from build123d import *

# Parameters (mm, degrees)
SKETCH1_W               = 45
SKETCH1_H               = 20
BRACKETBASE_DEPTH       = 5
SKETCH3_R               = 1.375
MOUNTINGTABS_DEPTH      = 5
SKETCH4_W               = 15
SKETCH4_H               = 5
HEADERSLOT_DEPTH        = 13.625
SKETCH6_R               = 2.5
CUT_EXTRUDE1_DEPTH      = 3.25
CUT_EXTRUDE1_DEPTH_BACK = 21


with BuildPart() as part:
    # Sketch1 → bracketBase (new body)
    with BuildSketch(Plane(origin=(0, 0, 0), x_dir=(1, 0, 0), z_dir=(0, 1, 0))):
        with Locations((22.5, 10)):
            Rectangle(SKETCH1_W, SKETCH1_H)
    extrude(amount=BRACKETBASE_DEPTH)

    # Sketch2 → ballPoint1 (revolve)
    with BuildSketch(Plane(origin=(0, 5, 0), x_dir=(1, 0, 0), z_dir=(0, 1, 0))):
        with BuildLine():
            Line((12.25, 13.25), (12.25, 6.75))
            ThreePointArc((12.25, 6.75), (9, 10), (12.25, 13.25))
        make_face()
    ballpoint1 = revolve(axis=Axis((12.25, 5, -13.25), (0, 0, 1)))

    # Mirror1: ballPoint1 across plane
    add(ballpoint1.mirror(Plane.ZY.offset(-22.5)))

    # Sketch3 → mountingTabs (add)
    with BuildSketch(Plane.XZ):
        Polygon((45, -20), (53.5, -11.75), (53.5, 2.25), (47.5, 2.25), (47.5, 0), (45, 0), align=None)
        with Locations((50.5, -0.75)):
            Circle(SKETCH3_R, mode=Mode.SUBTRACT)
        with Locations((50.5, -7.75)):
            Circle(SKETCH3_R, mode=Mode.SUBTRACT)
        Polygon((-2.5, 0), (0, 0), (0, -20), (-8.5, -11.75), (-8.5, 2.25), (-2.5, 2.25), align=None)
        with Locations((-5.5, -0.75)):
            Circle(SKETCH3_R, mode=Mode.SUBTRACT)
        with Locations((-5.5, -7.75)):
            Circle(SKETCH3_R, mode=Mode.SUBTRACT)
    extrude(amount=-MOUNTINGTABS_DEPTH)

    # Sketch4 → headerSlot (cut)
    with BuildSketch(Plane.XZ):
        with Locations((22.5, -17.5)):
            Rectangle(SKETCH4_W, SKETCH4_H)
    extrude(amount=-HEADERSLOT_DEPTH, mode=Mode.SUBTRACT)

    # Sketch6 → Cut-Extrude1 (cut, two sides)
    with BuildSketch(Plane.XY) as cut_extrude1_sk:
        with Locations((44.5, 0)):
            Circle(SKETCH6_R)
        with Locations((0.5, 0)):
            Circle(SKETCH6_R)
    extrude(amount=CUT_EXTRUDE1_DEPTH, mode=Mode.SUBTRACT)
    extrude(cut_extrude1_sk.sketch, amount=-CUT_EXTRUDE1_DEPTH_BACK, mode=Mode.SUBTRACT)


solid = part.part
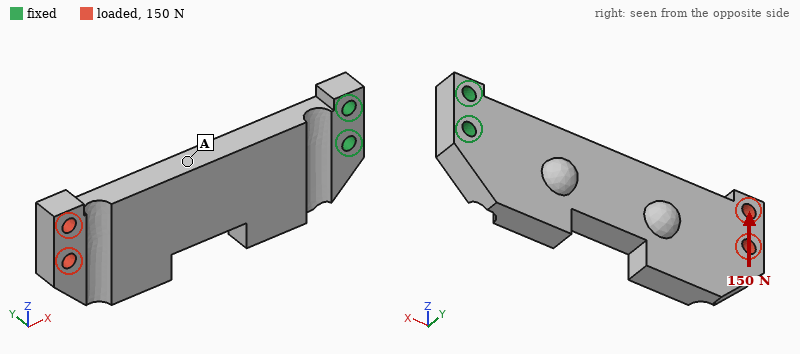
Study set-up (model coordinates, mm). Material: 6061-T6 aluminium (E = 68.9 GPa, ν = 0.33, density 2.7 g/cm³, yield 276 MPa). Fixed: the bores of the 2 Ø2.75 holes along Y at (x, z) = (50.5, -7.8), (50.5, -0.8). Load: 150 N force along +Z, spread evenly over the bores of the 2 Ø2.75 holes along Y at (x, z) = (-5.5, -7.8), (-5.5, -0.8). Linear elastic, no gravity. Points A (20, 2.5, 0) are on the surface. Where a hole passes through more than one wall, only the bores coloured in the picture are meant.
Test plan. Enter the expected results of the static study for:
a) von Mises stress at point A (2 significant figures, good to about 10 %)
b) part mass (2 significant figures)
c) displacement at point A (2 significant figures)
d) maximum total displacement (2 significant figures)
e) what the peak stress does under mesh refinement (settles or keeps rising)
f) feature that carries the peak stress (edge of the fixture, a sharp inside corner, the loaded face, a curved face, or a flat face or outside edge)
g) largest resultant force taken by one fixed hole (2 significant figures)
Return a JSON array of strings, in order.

["20 MPa", "14 g", "0.058 mm", "0.14 mm", "keeps rising", "edge of the fixture", "920 N"]
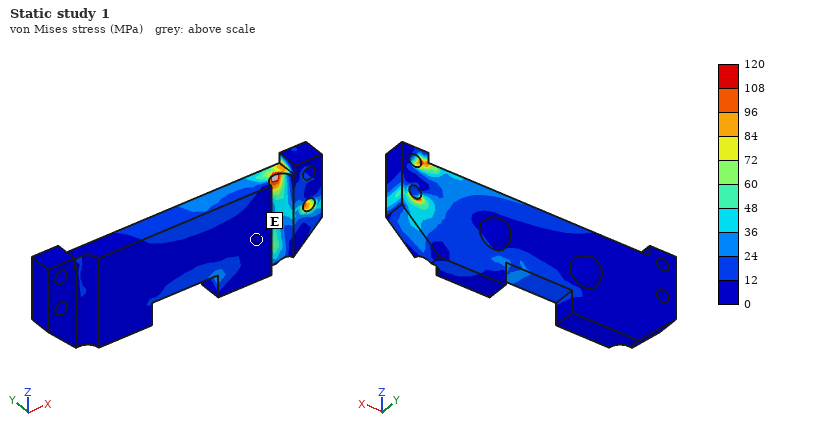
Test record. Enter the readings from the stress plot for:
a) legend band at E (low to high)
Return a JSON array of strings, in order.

["0 to 12 MPa"]
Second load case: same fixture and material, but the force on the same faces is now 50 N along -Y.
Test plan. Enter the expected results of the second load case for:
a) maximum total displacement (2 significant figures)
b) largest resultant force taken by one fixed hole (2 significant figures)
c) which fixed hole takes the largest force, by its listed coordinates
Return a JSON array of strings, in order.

["0.54 mm", "40 N", "(50.5, -7.8)"]
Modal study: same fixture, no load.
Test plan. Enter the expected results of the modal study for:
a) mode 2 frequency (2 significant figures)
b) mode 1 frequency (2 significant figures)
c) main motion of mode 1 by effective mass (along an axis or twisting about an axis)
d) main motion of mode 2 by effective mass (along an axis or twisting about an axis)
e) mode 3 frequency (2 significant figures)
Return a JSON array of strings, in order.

["2700 Hz", "790 Hz", "along Y", "along Z", "5400 Hz"]
